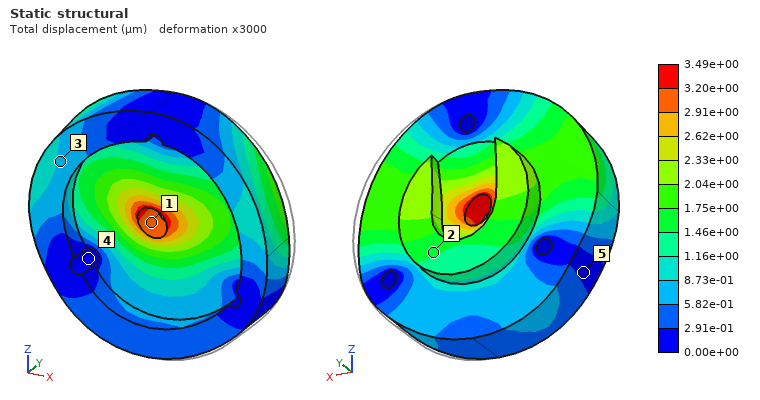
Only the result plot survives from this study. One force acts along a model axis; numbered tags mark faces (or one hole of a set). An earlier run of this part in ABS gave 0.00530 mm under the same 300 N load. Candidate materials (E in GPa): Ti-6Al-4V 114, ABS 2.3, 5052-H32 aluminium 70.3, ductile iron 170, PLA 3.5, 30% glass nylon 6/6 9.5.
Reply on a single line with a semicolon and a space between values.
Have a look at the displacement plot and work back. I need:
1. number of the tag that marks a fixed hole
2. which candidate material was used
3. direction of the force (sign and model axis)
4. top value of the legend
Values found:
4; PLA; -X; 3.49e+00 µm
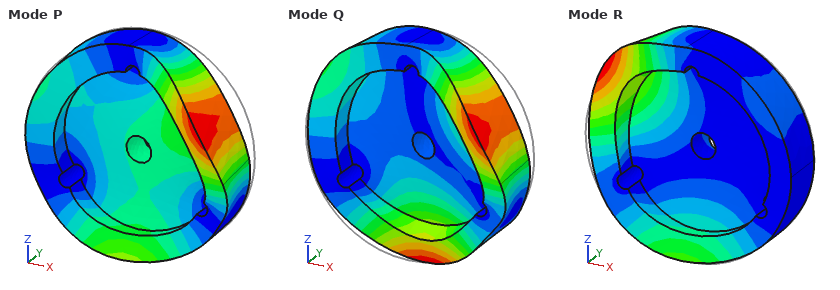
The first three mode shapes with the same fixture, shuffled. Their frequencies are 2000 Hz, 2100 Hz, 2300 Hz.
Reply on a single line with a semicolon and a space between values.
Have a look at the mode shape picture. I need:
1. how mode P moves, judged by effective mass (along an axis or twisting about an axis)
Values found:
along Y
